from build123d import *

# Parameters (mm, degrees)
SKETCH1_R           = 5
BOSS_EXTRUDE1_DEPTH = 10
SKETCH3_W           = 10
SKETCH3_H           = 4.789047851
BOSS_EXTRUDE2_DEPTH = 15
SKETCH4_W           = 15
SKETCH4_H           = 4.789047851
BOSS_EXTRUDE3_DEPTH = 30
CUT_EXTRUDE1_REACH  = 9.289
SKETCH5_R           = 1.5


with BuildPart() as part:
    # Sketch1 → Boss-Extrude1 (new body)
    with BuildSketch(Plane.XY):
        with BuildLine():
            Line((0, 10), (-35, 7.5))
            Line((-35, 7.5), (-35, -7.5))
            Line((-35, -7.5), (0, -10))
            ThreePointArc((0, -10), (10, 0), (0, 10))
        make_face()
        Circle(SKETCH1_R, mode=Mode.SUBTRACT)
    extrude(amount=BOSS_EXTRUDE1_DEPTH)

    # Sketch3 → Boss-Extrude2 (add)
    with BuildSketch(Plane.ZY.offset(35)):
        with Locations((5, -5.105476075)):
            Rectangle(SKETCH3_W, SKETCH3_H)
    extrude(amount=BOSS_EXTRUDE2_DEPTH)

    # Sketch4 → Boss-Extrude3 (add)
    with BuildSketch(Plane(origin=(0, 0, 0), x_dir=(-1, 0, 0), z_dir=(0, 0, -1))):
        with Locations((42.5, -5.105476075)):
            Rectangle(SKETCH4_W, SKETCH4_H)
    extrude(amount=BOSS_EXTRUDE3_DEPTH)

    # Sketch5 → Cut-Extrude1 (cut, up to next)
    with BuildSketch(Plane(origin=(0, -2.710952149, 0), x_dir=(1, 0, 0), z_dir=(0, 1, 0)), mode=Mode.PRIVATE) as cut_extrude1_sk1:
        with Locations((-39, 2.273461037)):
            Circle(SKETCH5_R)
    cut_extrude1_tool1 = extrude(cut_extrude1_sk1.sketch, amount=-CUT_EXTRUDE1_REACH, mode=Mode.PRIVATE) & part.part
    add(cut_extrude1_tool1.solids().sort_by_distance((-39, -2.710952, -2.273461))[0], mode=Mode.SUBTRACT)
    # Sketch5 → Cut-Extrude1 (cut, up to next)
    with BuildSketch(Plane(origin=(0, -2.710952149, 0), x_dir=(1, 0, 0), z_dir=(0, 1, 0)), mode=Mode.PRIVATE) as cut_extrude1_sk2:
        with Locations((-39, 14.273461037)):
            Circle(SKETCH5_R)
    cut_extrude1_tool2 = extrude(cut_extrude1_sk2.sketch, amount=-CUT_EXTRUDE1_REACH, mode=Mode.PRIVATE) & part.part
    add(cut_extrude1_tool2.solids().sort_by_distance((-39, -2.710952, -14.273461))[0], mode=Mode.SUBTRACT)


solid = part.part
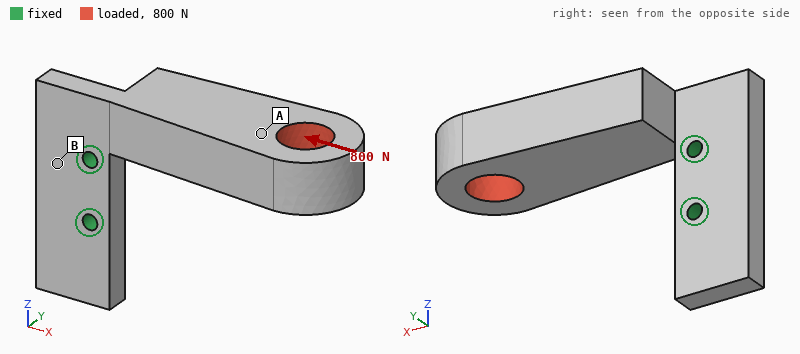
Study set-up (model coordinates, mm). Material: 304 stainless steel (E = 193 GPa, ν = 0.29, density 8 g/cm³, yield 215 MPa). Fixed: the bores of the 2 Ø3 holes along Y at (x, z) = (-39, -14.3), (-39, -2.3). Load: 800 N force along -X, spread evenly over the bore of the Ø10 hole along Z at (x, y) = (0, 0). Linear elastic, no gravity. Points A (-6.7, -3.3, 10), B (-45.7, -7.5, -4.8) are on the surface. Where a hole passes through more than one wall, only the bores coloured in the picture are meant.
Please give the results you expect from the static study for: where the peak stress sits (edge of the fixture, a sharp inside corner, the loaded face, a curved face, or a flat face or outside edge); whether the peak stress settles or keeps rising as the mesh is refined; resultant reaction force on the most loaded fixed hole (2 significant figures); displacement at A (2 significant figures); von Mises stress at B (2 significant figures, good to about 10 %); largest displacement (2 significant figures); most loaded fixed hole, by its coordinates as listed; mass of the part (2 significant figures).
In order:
edge of the fixture
keeps rising
1.1 kN
62 µm
30 MPa
97 µm
(-39, -2.3)
78 g
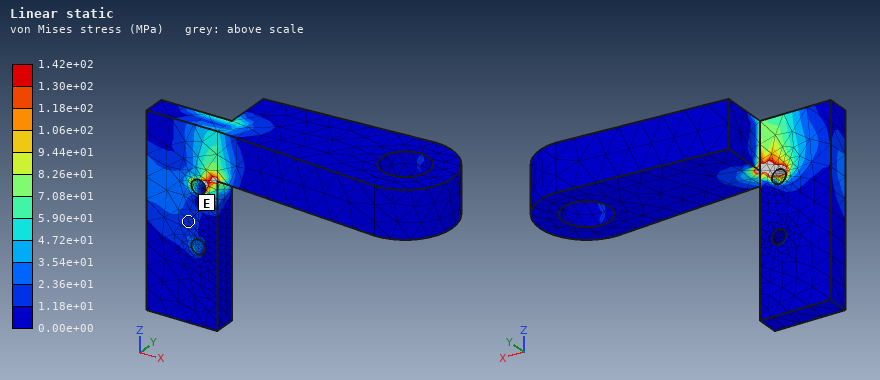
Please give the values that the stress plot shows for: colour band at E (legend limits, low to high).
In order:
1.18e+01 to 2.36e+01 MPa
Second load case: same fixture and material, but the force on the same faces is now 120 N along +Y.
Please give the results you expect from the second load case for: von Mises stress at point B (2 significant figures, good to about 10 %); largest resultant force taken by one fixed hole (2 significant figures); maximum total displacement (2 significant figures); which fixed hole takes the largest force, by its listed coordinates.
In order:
19 MPa
120 N
0.11 mm
(-39, -2.3)
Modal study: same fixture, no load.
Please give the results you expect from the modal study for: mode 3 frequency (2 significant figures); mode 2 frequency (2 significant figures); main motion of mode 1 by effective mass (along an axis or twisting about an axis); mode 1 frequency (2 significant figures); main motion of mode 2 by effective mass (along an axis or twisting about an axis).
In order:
4700 Hz
1900 Hz
along Y
1100 Hz
along Z
